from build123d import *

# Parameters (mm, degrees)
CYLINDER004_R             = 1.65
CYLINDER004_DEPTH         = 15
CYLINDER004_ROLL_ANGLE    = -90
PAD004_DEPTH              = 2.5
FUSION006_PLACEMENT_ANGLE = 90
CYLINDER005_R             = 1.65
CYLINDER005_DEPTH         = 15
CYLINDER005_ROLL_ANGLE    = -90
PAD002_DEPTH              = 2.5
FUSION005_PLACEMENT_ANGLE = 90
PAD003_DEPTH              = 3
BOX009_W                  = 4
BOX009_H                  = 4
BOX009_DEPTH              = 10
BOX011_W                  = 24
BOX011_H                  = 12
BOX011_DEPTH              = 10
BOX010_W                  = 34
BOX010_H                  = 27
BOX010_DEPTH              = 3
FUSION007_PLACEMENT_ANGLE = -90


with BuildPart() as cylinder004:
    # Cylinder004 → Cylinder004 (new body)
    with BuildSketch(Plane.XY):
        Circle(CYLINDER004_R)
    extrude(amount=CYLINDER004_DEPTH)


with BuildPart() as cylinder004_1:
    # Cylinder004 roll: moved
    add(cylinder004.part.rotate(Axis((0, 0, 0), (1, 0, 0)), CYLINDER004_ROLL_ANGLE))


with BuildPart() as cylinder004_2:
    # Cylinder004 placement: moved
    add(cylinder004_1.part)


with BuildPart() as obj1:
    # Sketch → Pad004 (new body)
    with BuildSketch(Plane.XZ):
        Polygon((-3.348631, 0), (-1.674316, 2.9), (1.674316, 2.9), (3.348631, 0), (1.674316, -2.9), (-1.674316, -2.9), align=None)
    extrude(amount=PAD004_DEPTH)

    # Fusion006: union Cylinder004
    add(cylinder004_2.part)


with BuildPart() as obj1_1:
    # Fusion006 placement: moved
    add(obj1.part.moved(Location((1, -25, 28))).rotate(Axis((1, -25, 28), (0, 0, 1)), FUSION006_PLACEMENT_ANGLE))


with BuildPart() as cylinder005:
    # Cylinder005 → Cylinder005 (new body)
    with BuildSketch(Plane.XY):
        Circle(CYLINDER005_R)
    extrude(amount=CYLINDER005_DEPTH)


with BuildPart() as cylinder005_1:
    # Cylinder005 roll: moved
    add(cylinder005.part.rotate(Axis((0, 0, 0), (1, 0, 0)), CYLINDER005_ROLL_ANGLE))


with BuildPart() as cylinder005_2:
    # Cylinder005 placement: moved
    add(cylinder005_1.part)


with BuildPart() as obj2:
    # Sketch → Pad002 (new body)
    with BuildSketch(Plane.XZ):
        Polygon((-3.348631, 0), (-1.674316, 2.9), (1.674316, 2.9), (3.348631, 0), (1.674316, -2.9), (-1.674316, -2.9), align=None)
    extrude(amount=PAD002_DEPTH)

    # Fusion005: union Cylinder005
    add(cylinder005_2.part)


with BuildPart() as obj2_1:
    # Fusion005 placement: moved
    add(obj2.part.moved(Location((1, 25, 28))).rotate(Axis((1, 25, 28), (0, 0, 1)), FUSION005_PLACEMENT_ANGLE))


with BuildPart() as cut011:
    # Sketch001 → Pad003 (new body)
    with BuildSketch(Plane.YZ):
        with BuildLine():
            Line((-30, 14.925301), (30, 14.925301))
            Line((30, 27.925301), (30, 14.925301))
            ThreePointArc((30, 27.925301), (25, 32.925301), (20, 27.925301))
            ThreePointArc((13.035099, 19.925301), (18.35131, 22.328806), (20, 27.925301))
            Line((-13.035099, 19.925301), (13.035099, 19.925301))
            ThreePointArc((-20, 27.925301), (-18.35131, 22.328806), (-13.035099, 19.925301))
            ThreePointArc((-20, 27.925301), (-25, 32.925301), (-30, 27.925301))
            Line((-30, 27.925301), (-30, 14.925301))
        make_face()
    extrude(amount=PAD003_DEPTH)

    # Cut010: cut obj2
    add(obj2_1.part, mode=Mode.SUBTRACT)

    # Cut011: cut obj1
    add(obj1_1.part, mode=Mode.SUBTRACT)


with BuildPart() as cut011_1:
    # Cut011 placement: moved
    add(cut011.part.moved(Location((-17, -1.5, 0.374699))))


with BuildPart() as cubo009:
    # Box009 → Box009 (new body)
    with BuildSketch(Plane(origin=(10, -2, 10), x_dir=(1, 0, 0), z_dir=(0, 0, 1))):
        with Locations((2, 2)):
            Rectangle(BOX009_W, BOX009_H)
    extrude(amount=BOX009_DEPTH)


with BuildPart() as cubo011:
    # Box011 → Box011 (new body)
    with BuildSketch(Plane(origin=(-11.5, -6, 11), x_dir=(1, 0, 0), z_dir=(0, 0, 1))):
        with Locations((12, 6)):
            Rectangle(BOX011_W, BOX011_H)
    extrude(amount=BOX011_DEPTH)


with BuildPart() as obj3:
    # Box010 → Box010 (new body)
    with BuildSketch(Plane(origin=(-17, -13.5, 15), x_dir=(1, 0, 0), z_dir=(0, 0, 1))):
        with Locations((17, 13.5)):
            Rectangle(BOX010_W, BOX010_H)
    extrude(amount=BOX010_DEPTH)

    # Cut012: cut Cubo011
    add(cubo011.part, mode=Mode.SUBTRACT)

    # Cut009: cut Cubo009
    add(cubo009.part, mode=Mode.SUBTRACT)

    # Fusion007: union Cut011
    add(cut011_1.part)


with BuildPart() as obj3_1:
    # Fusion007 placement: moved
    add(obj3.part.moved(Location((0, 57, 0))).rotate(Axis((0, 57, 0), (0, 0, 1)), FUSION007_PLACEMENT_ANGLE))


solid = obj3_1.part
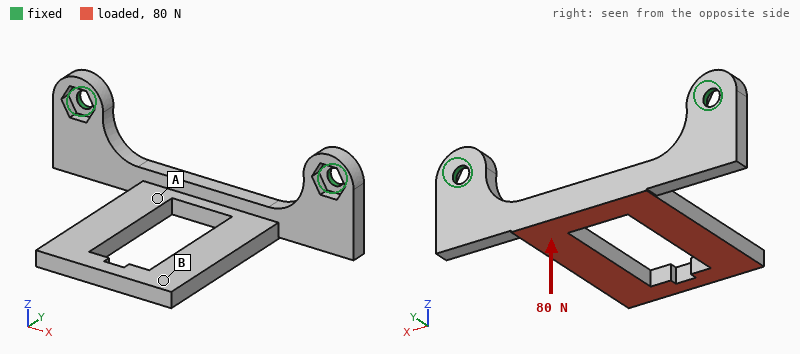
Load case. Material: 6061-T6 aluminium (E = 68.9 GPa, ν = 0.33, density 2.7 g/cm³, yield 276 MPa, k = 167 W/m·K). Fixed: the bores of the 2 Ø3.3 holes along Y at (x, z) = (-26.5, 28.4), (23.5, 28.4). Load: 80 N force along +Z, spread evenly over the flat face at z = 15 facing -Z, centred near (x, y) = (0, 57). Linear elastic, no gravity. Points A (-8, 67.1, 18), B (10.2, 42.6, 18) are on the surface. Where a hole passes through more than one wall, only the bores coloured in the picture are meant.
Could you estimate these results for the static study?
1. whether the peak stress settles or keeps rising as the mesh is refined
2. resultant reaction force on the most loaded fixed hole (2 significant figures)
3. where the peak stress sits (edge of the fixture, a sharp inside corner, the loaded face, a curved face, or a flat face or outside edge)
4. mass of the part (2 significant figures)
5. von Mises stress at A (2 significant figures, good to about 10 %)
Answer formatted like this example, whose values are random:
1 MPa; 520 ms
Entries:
keeps rising; 62 N; edge of the fixture; 8.6 g; 37 MPa
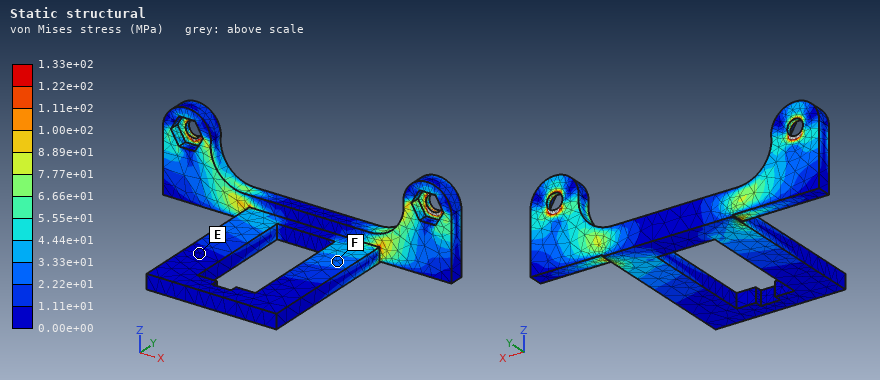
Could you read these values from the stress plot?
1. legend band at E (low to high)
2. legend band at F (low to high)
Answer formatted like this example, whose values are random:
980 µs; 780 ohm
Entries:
0.00e+00 to 1.11e+01 MPa; 2.22e+01 to 3.33e+01 MPa
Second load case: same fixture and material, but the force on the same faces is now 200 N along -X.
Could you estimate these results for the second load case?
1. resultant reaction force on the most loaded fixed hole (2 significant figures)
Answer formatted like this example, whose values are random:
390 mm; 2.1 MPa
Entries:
130 N
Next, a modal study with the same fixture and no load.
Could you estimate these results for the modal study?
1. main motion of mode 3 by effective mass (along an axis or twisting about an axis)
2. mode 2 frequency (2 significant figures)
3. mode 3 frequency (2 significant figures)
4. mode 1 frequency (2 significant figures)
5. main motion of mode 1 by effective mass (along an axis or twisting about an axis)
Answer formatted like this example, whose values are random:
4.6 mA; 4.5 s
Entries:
along Y; 2700 Hz; 3000 Hz; 980 Hz; along Z
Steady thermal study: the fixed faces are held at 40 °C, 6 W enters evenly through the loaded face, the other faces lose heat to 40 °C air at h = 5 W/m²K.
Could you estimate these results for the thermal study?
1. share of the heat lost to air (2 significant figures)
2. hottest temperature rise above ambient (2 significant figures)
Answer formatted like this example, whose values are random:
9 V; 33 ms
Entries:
3.1 %; 29 K
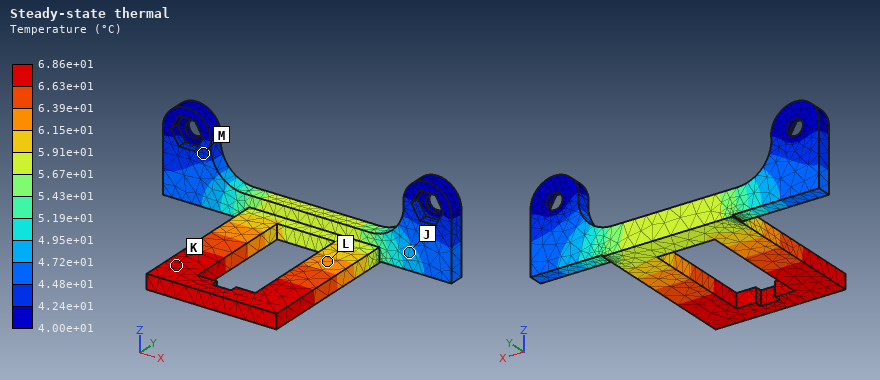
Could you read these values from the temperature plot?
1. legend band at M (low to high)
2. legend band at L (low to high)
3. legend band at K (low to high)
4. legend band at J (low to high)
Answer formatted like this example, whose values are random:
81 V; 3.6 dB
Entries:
4.24e+01 to 4.48e+01 °C; 6.15e+01 to 6.39e+01 °C; 6.63e+01 to 6.86e+01 °C; 4.72e+01 to 4.95e+01 °C
